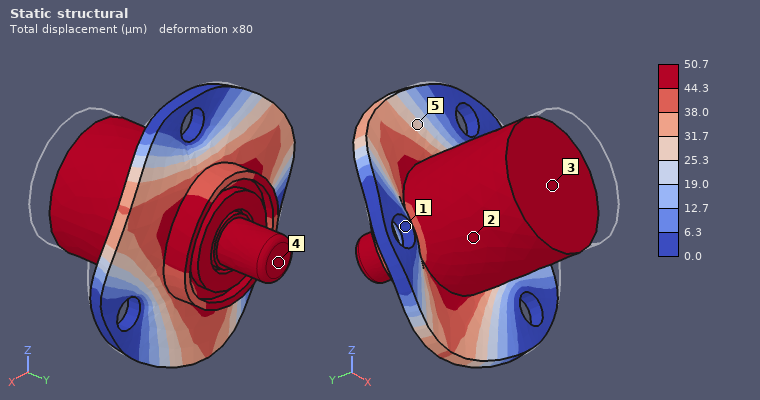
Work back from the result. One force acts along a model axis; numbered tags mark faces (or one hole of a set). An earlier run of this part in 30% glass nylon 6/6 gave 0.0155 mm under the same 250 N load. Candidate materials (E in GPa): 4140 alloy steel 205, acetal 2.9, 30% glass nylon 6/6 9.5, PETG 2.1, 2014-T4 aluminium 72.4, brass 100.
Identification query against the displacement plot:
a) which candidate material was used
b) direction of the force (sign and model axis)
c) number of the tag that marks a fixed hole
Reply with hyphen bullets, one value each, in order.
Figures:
- acetal
- +Y
- 1
